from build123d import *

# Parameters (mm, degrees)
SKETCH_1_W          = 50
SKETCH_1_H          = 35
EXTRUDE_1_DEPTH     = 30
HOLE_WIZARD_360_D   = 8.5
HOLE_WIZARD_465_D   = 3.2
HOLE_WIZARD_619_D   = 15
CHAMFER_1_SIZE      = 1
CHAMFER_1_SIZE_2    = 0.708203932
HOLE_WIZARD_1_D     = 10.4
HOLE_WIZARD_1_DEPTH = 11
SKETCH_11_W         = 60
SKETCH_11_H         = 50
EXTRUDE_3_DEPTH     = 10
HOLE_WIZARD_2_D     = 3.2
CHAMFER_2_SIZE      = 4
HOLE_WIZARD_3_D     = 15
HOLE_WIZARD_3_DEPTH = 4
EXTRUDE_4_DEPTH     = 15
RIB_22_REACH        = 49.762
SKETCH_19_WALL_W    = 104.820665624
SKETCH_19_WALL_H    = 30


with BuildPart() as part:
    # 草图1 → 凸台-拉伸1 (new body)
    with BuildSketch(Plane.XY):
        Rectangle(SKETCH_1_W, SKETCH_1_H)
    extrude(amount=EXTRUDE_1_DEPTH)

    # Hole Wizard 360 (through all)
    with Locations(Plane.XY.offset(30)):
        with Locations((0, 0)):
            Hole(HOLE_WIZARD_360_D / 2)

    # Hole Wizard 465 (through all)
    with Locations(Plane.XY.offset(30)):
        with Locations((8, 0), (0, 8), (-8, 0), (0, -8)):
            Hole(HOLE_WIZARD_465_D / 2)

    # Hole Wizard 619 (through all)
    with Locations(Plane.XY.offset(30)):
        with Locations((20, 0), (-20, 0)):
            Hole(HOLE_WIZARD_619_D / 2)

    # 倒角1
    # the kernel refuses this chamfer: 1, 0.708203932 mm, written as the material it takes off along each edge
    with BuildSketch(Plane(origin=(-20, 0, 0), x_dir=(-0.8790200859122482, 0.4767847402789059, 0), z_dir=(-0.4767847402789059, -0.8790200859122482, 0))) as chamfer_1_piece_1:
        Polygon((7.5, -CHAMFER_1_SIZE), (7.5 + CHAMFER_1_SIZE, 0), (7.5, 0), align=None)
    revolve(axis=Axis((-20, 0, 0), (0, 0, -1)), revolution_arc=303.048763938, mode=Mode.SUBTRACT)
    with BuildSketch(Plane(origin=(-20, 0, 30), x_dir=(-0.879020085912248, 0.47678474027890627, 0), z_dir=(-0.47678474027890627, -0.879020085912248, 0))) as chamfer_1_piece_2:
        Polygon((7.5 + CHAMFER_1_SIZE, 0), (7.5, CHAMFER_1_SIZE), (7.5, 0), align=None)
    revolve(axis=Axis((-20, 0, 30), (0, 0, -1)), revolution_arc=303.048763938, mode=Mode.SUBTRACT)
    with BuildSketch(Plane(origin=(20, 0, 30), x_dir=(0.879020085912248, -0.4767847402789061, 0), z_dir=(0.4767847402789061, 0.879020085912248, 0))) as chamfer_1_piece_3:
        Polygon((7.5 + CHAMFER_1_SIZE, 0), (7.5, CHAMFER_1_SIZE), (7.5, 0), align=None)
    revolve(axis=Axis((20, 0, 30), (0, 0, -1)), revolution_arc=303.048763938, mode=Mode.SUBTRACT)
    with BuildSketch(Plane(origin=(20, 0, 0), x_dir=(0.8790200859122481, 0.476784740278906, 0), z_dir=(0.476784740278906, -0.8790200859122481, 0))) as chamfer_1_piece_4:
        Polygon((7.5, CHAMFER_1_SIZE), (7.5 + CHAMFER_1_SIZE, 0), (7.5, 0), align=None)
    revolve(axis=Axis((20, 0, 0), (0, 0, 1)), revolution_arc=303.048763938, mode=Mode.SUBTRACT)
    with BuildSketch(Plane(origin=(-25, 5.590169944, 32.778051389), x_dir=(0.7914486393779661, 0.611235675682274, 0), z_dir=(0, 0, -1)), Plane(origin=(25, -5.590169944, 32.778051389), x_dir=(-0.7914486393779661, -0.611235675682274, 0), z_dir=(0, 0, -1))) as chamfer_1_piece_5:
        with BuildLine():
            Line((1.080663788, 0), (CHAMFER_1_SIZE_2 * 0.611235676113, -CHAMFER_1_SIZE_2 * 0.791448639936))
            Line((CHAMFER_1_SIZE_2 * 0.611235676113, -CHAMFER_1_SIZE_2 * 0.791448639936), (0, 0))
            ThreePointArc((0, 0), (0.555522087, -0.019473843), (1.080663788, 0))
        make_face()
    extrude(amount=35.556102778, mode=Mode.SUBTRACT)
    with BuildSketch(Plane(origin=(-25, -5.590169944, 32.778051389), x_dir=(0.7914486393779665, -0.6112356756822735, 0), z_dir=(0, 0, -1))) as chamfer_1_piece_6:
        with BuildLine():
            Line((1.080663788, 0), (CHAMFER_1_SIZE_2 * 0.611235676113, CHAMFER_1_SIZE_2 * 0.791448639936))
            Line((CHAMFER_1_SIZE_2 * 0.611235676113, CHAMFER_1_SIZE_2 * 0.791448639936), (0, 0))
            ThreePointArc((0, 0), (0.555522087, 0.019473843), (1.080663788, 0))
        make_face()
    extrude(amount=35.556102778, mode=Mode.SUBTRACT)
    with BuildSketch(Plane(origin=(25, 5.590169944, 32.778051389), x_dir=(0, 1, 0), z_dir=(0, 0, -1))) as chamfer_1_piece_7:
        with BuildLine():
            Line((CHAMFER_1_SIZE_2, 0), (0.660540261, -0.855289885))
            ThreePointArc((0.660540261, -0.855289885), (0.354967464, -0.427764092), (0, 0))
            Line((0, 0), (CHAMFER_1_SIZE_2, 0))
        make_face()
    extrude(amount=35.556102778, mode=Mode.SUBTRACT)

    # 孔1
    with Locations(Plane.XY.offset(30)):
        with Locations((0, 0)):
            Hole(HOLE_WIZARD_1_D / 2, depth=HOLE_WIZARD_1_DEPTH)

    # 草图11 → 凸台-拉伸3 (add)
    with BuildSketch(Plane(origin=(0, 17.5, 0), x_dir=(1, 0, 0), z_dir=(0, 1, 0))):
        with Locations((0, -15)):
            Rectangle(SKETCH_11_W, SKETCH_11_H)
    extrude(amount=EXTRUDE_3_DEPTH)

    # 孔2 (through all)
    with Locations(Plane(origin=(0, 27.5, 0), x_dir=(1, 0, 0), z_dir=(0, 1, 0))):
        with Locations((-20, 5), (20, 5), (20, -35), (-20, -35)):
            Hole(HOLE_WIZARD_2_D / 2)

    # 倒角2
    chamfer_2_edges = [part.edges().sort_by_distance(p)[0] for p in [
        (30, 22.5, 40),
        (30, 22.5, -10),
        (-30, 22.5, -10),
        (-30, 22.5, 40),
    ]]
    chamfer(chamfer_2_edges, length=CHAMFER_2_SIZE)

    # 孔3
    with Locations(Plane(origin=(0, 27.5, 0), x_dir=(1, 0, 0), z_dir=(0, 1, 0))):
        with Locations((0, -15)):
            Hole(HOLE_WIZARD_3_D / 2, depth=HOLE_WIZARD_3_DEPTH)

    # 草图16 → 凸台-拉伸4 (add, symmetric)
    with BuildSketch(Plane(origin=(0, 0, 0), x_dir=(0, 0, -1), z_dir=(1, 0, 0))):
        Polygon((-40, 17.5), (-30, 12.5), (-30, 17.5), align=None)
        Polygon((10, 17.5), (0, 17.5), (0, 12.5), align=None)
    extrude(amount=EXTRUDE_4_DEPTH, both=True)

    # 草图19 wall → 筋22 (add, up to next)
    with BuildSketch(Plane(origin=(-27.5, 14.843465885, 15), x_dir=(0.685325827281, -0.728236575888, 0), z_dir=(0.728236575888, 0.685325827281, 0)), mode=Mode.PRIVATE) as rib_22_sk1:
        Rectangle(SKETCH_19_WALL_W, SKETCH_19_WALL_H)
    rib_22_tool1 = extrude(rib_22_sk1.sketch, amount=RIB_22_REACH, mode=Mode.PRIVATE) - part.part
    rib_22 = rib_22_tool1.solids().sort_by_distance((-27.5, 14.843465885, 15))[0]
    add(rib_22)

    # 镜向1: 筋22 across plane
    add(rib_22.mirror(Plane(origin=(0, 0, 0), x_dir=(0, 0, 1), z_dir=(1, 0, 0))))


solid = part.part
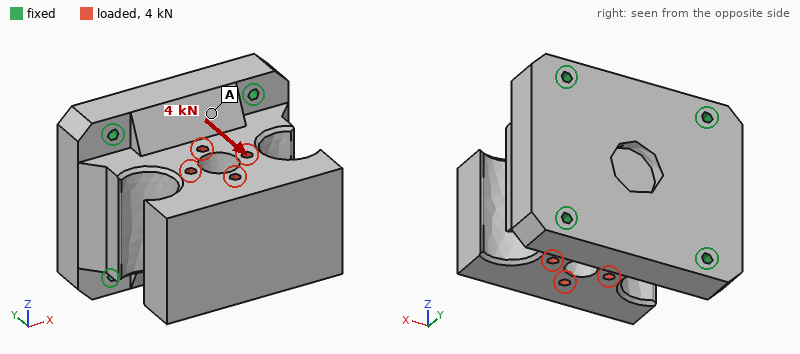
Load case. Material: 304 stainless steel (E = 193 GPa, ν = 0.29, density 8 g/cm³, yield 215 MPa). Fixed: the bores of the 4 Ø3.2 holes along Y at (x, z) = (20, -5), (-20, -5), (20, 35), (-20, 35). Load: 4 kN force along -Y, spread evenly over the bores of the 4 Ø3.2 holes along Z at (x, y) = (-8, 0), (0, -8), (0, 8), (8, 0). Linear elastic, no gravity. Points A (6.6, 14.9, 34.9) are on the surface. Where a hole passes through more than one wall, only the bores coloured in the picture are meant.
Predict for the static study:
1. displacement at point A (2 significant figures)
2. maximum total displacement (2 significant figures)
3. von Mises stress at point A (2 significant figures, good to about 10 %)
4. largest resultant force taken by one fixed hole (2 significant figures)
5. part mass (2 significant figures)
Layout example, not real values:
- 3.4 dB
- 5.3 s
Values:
- 1.1 µm
- 2.0 µm
- 4.9 MPa
- 1.1 kN
- 570 g
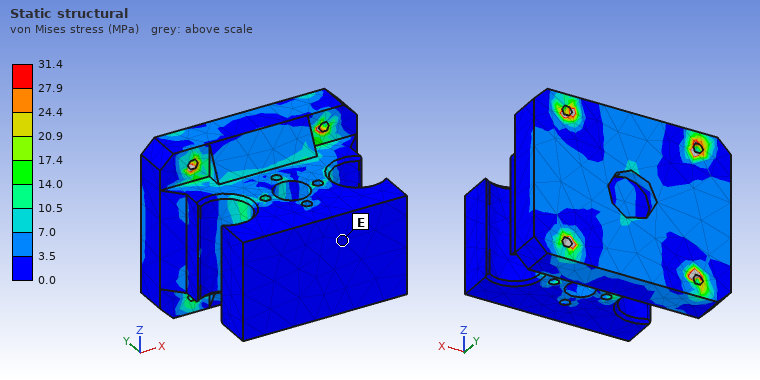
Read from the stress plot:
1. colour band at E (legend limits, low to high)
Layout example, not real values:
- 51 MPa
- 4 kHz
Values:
- 0.0 to 3.5 MPa
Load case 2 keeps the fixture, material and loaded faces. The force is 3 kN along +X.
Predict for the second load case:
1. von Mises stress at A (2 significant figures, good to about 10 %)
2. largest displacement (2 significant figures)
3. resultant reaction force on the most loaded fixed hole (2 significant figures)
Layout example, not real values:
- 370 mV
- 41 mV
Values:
- 6.0 MPa
- 4.3 µm
- 1.1 kN
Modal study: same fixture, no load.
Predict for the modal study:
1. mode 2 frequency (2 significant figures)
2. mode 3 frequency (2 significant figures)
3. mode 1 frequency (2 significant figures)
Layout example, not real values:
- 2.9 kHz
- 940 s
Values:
- 8000 Hz
- 11 kHz
- 7700 Hz
